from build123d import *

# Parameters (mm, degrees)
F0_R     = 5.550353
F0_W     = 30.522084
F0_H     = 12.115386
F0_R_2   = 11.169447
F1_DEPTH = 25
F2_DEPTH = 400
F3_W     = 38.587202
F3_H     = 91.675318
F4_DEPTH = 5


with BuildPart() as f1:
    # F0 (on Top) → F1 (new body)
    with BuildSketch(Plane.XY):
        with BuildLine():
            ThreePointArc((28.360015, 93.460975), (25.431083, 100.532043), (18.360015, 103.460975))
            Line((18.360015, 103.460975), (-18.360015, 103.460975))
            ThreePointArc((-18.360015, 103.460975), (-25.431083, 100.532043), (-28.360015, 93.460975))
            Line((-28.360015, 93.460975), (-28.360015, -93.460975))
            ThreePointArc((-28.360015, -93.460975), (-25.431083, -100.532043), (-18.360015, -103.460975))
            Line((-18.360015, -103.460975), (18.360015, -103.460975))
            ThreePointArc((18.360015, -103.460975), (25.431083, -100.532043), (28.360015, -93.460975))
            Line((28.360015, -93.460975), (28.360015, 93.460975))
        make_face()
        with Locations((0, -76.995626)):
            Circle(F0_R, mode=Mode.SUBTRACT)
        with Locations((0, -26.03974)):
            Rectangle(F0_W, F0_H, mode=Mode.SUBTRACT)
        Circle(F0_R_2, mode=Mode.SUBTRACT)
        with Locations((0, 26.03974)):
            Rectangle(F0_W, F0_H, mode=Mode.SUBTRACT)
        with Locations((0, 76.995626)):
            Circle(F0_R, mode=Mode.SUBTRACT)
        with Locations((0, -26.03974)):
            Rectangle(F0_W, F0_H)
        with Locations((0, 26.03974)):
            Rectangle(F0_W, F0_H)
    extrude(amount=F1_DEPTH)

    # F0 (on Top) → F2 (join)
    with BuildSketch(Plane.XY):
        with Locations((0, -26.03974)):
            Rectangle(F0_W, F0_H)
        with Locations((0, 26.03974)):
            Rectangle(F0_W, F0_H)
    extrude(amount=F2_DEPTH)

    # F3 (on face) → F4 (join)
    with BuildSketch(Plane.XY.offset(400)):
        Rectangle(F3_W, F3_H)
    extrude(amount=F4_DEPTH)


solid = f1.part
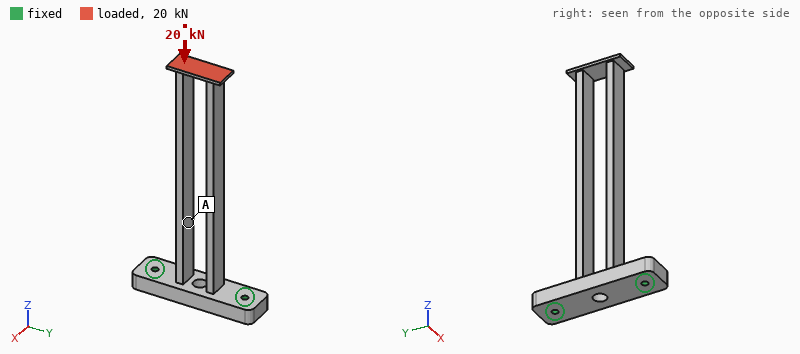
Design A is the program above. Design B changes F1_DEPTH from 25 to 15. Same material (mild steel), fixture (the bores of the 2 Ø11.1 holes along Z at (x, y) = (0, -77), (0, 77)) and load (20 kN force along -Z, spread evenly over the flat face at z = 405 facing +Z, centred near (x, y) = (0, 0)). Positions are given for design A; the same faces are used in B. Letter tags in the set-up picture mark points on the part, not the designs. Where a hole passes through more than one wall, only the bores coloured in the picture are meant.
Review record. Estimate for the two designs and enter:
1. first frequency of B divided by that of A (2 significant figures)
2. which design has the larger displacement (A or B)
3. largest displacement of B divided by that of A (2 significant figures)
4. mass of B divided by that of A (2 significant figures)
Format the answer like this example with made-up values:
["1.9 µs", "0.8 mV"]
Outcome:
["0.93", "B", "1.5", "0.82"]
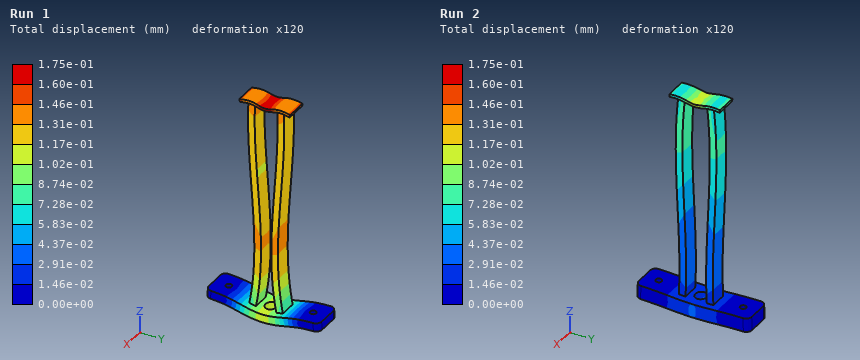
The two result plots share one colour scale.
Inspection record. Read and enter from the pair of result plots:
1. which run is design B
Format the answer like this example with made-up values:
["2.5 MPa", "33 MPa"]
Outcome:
["Run 1"]
